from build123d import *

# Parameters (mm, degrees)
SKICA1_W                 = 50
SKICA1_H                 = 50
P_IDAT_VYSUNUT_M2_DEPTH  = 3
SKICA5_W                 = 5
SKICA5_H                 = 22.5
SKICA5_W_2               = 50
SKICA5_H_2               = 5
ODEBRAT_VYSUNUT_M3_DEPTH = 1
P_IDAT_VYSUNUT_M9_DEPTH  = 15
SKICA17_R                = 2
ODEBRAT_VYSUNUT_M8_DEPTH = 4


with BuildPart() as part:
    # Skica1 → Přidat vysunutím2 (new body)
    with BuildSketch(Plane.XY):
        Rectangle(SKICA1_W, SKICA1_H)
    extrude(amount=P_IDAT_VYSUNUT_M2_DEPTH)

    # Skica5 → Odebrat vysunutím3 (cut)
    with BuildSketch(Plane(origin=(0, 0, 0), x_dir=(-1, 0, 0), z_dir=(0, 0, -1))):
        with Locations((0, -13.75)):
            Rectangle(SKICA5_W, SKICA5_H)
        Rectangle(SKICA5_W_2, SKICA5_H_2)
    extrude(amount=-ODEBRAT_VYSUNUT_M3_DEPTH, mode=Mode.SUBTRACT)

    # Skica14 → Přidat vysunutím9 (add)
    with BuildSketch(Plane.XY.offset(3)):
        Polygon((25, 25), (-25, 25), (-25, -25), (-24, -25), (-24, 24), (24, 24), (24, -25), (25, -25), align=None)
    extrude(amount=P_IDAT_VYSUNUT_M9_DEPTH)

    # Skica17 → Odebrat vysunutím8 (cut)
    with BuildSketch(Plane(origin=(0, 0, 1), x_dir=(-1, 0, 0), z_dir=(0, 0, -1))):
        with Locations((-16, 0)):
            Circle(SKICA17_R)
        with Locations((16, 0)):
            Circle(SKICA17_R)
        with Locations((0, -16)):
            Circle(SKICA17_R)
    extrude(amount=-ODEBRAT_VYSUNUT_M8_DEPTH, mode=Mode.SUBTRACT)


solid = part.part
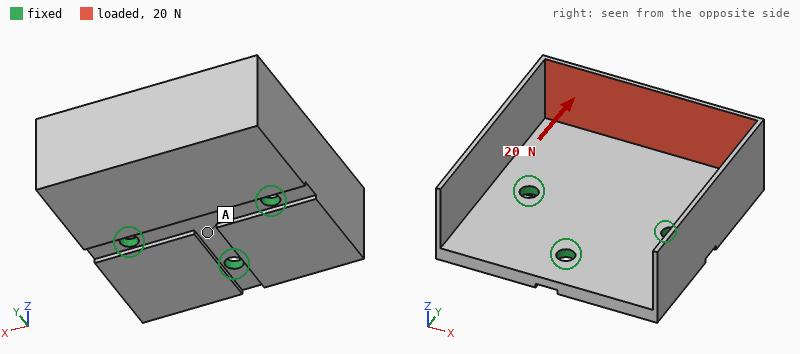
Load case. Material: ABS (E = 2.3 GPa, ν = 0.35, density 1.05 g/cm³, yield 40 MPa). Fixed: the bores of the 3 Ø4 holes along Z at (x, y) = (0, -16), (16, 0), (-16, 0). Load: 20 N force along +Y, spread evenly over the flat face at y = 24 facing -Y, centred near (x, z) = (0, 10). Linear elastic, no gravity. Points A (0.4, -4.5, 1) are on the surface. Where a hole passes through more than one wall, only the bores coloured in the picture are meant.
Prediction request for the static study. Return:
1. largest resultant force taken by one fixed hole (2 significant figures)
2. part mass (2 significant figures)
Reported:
10 N
9.7 g
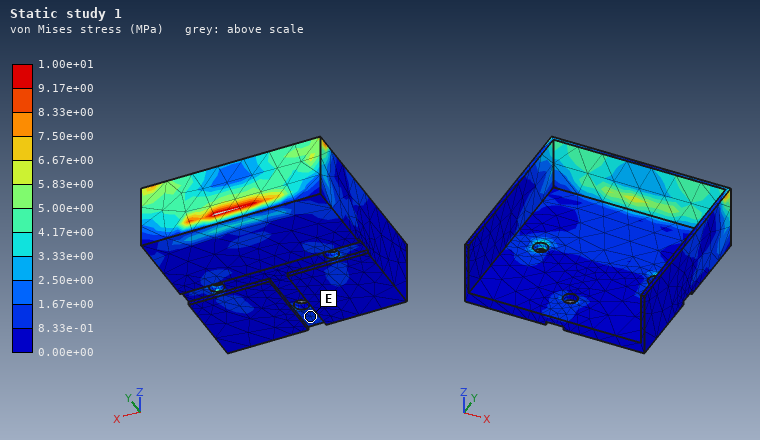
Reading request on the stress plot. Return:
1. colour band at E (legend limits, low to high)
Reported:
8.33e-01 to 1.67e+00 MPa
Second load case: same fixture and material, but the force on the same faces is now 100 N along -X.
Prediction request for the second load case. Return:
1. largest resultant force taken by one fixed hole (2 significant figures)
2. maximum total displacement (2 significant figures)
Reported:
89 N
0.77 mm
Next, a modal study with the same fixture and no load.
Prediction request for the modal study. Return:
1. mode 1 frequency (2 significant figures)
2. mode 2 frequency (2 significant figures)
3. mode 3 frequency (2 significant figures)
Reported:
780 Hz
990 Hz
1100 Hz
